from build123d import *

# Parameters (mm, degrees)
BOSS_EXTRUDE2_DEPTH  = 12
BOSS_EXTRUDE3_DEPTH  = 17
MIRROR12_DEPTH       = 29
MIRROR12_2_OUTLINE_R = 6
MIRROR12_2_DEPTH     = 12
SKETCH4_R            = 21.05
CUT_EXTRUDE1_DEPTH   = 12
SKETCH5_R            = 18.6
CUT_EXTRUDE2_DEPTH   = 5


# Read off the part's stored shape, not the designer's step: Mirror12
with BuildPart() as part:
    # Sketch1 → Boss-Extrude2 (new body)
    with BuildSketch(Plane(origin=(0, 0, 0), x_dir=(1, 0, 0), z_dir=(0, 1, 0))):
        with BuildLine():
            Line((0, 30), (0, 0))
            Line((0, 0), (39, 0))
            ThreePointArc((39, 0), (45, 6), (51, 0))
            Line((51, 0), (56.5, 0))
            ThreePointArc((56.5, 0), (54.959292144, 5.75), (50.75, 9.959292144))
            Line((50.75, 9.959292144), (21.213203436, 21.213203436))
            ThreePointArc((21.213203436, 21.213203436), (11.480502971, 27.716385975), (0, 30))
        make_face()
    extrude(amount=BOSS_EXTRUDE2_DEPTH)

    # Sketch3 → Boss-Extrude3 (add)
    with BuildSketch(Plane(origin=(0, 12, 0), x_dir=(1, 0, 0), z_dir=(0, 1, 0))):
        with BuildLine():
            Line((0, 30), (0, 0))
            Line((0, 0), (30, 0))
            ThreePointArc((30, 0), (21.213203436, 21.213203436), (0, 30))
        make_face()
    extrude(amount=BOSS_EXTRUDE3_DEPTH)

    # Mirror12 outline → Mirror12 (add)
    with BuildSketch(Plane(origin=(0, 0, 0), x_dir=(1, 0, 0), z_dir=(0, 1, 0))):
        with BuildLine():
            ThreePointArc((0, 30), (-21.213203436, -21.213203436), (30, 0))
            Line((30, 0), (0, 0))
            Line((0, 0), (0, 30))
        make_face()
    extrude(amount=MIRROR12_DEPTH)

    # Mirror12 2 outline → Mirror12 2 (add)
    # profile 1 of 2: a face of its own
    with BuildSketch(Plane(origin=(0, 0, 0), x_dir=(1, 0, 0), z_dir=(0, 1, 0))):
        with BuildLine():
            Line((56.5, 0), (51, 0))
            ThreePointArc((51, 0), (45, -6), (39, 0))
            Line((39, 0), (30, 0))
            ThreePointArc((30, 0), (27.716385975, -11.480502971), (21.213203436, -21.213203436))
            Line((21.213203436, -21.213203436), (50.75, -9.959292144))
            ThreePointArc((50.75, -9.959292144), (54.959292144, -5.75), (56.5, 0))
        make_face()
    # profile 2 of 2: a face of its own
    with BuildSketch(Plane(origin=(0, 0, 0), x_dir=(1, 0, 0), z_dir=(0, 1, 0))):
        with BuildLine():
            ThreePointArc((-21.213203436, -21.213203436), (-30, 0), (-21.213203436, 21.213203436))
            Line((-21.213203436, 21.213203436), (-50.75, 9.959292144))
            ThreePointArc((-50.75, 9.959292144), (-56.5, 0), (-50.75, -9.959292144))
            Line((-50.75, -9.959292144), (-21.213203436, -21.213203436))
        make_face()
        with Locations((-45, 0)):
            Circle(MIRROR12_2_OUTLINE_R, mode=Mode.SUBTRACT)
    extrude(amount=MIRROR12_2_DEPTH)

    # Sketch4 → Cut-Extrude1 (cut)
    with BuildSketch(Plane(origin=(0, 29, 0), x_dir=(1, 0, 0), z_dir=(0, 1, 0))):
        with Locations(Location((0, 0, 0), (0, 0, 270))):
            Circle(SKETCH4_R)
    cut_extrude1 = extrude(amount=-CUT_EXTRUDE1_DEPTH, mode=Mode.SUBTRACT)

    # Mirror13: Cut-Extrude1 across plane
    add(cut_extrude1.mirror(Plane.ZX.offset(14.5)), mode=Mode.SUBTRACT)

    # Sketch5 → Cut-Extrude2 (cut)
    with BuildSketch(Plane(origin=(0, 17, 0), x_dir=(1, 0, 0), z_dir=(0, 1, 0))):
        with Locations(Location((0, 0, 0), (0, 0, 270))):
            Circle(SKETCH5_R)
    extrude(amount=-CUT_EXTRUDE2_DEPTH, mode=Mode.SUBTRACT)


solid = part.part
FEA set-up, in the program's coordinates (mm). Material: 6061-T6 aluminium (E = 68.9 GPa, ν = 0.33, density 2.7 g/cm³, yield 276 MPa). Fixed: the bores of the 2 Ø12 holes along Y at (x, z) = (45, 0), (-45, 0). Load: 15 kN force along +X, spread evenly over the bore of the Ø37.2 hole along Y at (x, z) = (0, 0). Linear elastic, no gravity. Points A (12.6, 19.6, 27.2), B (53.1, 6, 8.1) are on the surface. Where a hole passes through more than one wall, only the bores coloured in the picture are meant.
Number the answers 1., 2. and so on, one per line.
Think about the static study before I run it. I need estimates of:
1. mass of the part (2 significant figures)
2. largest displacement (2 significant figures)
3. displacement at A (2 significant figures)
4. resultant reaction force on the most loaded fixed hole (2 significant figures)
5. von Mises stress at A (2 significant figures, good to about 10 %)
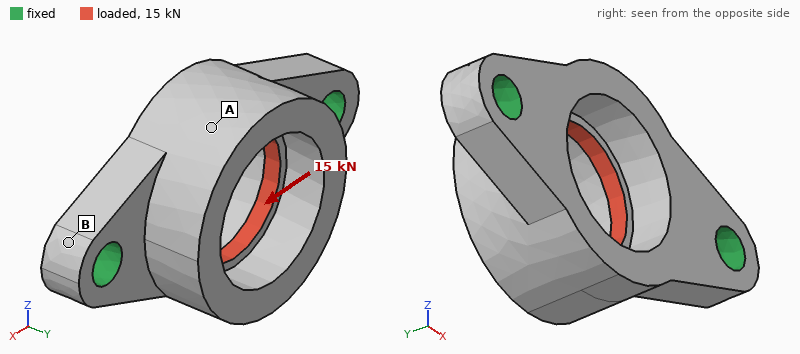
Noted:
1. 160 g
2. 18 µm
3. 14 µm
4. 7.7 kN
5. 9.4 MPa
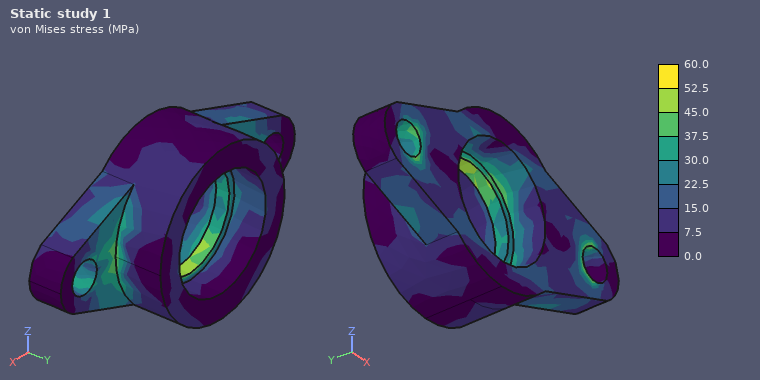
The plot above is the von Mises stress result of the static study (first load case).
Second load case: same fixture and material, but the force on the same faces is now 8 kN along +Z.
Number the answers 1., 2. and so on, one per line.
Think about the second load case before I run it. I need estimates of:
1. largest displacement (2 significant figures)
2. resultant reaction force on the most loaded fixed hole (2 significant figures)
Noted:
1. 64 µm
2. 4.0 kN
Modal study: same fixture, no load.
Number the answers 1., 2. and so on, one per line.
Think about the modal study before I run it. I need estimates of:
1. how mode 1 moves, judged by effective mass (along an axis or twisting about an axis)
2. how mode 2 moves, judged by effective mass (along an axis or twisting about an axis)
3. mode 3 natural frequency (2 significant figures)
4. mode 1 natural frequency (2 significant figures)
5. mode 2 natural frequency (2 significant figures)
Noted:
1. along Z
2. along Y
3. 11 kHz
4. 4600 Hz
5. 6700 Hz
